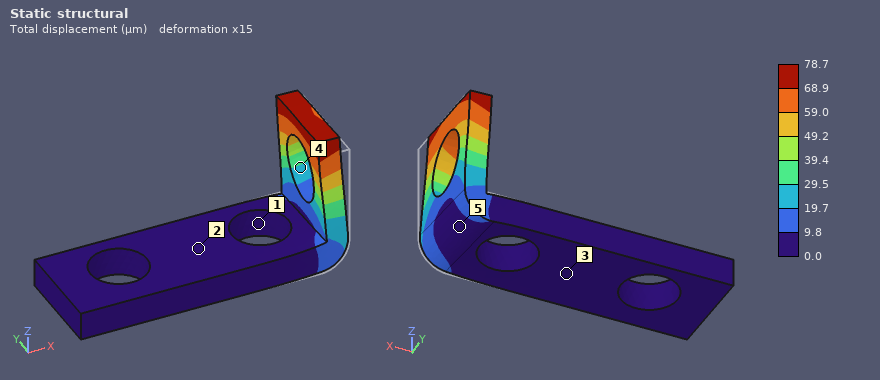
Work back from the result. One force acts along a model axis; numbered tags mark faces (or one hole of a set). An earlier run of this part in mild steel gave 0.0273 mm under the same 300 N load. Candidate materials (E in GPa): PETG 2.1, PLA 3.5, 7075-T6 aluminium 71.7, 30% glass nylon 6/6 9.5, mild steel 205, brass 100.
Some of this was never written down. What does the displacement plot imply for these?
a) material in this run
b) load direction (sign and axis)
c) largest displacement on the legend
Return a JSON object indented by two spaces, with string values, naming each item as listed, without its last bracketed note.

{
  "material in this run": "7075-T6 aluminium",
  "load direction": "+Y",
  "largest displacement on the legend": "78.7 µm"
}
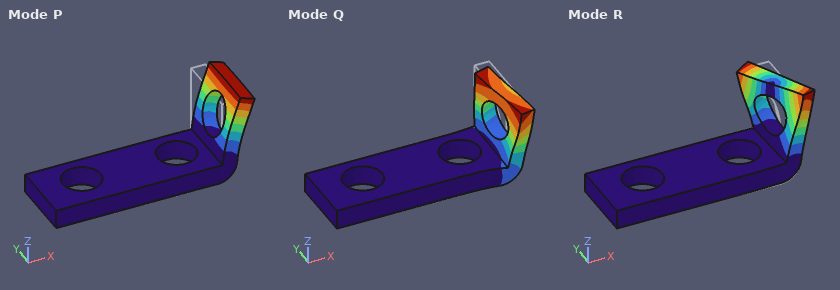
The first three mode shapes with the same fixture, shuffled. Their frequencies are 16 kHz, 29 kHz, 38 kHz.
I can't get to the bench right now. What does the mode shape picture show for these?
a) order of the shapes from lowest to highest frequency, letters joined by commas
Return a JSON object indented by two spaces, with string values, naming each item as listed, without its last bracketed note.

{
  "order of the shapes from lowest to highest frequency, letters joined by commas": "P, Q, R"
}
